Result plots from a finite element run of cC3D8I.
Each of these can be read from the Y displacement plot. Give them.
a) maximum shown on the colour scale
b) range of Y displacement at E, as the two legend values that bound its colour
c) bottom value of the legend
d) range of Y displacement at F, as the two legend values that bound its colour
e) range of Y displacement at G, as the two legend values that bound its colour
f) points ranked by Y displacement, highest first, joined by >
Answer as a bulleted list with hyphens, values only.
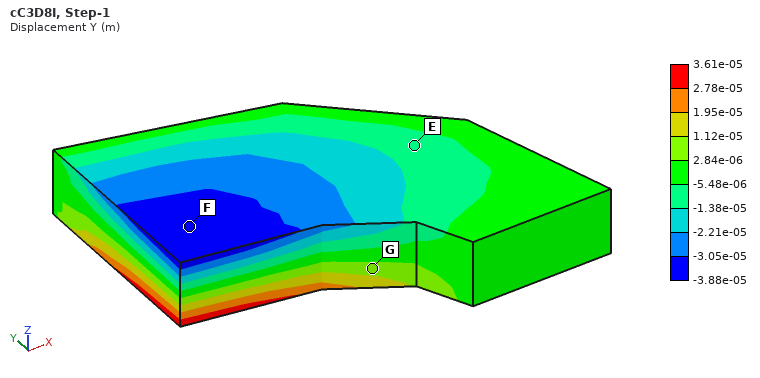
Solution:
- 3.61e-05 m
- -1.38e-05 to -5.48e-06 m
- -3.88e-05 m
- -3.88e-05 to -3.05e-05 m
- 2.84e-06 to 1.12e-05 m
- G > E > F
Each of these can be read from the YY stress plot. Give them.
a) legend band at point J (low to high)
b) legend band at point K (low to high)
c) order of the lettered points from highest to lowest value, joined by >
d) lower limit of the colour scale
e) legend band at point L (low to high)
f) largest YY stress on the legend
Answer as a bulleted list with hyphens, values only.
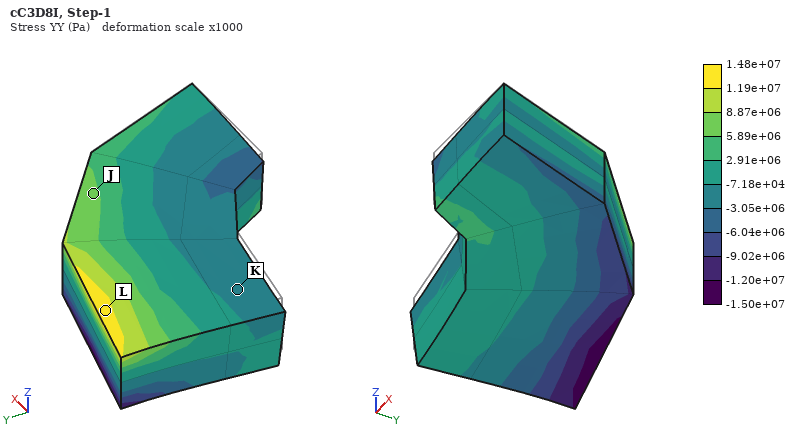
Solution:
- 5.89e+06 to 8.87e+06 Pa
- -3.05e+06 to -7.18e+04 Pa
- L > J > K
- -1.50e+07 Pa
- 1.19e+07 to 1.48e+07 Pa
- 1.48e+07 Pa
